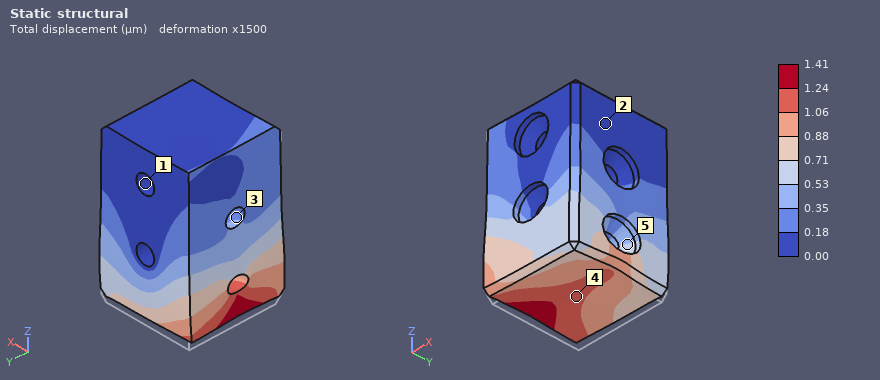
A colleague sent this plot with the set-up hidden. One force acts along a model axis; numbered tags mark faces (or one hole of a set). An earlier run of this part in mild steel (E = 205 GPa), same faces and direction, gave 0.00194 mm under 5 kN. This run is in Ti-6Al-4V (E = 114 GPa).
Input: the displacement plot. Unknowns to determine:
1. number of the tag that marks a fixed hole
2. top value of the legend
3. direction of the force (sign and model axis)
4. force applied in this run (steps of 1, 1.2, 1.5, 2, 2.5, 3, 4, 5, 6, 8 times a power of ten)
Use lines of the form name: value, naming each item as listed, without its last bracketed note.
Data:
number of the tag that marks a fixed hole: 1
top value of the legend: 1.41 µm
direction of the force: +Z
force applied in this run: 2 kN
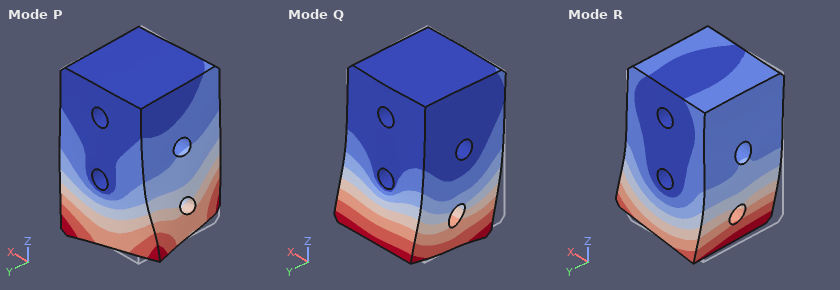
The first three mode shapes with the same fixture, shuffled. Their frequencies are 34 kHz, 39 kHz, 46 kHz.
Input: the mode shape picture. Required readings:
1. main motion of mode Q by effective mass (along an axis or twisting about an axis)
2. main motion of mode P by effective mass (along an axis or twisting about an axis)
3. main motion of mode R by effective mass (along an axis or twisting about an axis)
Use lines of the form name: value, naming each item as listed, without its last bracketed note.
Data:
main motion of mode Q by effective mass: along Y
main motion of mode P by effective mass: twisting about Z
main motion of mode R by effective mass: along X
